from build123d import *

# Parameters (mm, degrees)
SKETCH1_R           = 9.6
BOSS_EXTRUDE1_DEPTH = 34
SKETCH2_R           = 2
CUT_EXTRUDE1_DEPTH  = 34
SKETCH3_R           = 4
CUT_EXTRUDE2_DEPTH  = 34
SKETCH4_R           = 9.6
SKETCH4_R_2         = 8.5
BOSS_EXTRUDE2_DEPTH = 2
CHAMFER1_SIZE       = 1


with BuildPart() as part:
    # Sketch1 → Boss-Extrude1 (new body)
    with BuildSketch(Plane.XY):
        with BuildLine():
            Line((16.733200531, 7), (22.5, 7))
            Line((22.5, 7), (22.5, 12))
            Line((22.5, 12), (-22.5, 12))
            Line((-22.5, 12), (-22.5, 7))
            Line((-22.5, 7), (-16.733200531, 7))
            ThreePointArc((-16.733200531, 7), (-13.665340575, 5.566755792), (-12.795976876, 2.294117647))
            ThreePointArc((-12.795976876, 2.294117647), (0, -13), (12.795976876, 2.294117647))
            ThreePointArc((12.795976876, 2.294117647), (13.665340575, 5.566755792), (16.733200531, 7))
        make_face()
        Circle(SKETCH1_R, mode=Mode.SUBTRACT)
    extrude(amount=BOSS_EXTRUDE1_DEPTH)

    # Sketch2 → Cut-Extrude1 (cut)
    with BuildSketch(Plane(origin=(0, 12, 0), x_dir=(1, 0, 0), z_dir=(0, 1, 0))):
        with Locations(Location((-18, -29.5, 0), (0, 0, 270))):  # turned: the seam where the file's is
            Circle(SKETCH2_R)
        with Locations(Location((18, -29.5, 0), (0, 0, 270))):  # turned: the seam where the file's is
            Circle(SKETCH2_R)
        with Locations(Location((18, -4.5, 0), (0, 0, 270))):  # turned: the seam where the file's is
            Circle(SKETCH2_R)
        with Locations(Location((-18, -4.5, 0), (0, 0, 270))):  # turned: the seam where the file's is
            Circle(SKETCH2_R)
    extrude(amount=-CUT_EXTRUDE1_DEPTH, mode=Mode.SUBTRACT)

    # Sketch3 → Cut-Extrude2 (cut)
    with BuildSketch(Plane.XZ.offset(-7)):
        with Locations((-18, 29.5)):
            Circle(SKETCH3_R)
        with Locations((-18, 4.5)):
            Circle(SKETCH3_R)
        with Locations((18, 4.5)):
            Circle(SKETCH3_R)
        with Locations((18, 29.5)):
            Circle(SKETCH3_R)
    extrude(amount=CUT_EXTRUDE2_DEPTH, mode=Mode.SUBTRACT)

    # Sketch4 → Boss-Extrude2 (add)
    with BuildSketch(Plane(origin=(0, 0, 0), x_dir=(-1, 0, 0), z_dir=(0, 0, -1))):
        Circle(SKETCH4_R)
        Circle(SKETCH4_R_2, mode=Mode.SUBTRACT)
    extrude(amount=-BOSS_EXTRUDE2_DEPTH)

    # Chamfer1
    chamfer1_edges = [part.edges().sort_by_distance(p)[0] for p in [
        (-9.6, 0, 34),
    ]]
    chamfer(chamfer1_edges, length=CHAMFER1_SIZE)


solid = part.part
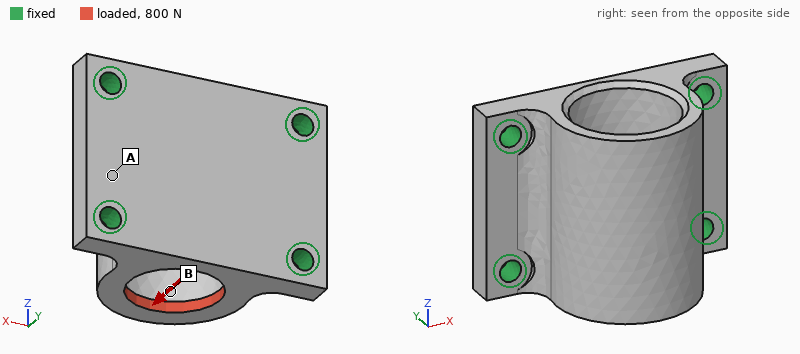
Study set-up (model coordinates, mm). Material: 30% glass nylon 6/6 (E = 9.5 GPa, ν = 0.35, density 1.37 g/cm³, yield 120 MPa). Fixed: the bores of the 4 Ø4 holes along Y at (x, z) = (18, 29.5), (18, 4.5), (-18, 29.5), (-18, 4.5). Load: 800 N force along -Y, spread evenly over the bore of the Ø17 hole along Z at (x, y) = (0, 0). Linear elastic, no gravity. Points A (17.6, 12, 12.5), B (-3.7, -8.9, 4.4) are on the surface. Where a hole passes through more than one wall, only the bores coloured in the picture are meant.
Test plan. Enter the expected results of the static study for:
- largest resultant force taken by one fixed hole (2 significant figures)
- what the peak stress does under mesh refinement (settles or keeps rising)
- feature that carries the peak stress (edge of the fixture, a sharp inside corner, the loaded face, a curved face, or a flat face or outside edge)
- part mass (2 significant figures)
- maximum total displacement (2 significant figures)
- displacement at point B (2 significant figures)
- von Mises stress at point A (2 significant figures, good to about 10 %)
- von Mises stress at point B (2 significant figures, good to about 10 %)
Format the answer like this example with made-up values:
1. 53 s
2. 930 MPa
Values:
1. 440 N
2. keeps rising
3. edge of the fixture
4. 18 g
5. 85 µm
6. 41 µm
7. 3.7 MPa
8. 6.9 MPa
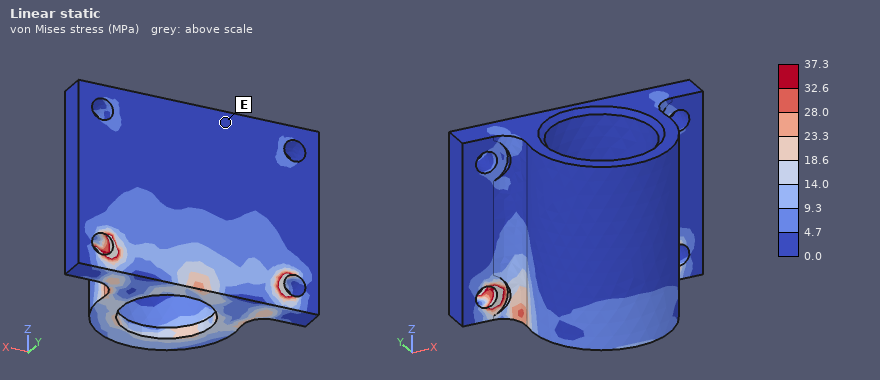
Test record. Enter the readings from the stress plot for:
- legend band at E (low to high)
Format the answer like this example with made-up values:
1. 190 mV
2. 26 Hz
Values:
1. 0.0 to 4.7 MPa
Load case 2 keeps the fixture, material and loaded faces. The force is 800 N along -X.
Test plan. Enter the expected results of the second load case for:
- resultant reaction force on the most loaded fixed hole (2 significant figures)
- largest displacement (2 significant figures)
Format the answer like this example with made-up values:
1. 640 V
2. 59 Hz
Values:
1. 320 N
2. 0.10 mm
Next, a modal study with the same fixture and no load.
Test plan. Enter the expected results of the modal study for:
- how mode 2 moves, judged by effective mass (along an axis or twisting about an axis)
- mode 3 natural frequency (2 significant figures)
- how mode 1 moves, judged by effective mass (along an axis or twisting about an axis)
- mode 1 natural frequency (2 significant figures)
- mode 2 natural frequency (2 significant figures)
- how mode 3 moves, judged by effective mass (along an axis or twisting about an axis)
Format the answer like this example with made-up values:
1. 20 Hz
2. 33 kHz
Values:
1. along Z
2. 8600 Hz
3. along X
4. 6300 Hz
5. 8000 Hz
6. along Y
